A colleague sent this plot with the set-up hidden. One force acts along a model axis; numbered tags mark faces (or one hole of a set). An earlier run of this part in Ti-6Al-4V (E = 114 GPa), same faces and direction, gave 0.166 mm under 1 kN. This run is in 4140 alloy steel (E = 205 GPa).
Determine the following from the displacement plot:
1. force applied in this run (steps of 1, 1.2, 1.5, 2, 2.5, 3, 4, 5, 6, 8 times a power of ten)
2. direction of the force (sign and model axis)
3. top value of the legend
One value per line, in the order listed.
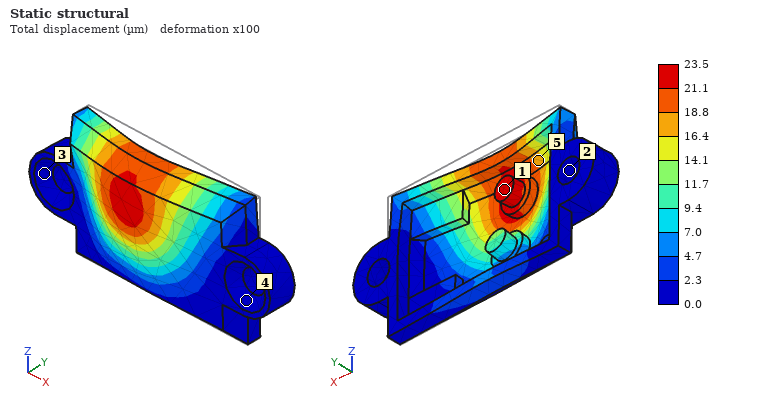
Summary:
250 N
-Y
23.5 µm
